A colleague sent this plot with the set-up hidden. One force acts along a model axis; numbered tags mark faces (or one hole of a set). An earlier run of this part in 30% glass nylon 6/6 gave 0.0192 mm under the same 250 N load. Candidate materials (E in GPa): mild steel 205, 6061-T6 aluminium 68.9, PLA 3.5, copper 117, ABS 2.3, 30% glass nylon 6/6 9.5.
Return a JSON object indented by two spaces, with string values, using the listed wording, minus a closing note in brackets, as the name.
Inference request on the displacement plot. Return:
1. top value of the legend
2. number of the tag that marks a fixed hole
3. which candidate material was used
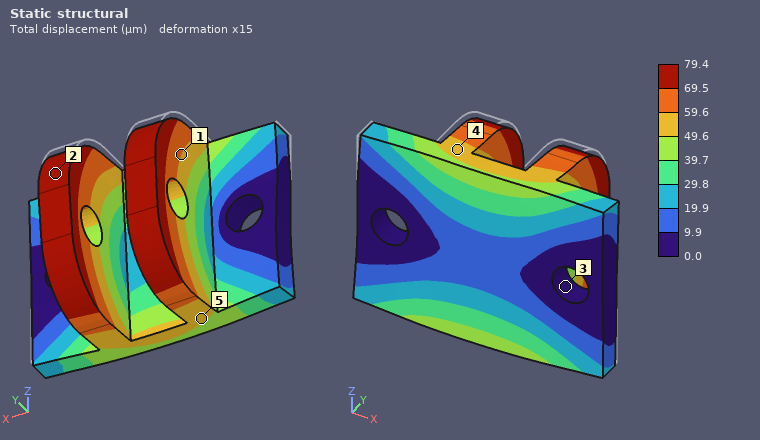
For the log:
{
  "top value of the legend": "79.4 µm",
  "number of the tag that marks a fixed hole": "3",
  "which candidate material was used": "ABS"
}
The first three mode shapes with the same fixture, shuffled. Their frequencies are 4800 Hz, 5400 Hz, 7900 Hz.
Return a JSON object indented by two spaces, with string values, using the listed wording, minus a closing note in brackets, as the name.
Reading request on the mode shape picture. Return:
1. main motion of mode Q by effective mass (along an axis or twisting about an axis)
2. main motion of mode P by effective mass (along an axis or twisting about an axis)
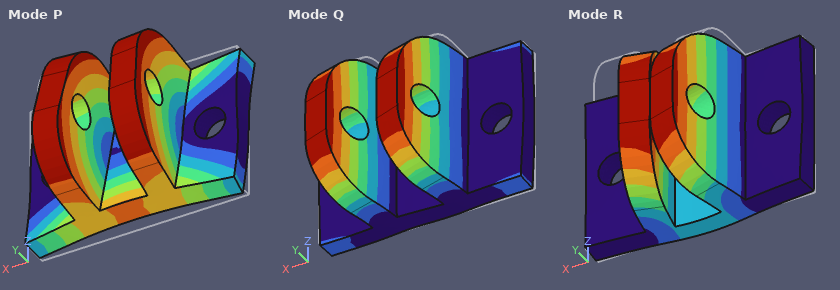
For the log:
{
  "main motion of mode Q by effective mass": "along X",
  "main motion of mode P by effective mass": "along Z"
}
